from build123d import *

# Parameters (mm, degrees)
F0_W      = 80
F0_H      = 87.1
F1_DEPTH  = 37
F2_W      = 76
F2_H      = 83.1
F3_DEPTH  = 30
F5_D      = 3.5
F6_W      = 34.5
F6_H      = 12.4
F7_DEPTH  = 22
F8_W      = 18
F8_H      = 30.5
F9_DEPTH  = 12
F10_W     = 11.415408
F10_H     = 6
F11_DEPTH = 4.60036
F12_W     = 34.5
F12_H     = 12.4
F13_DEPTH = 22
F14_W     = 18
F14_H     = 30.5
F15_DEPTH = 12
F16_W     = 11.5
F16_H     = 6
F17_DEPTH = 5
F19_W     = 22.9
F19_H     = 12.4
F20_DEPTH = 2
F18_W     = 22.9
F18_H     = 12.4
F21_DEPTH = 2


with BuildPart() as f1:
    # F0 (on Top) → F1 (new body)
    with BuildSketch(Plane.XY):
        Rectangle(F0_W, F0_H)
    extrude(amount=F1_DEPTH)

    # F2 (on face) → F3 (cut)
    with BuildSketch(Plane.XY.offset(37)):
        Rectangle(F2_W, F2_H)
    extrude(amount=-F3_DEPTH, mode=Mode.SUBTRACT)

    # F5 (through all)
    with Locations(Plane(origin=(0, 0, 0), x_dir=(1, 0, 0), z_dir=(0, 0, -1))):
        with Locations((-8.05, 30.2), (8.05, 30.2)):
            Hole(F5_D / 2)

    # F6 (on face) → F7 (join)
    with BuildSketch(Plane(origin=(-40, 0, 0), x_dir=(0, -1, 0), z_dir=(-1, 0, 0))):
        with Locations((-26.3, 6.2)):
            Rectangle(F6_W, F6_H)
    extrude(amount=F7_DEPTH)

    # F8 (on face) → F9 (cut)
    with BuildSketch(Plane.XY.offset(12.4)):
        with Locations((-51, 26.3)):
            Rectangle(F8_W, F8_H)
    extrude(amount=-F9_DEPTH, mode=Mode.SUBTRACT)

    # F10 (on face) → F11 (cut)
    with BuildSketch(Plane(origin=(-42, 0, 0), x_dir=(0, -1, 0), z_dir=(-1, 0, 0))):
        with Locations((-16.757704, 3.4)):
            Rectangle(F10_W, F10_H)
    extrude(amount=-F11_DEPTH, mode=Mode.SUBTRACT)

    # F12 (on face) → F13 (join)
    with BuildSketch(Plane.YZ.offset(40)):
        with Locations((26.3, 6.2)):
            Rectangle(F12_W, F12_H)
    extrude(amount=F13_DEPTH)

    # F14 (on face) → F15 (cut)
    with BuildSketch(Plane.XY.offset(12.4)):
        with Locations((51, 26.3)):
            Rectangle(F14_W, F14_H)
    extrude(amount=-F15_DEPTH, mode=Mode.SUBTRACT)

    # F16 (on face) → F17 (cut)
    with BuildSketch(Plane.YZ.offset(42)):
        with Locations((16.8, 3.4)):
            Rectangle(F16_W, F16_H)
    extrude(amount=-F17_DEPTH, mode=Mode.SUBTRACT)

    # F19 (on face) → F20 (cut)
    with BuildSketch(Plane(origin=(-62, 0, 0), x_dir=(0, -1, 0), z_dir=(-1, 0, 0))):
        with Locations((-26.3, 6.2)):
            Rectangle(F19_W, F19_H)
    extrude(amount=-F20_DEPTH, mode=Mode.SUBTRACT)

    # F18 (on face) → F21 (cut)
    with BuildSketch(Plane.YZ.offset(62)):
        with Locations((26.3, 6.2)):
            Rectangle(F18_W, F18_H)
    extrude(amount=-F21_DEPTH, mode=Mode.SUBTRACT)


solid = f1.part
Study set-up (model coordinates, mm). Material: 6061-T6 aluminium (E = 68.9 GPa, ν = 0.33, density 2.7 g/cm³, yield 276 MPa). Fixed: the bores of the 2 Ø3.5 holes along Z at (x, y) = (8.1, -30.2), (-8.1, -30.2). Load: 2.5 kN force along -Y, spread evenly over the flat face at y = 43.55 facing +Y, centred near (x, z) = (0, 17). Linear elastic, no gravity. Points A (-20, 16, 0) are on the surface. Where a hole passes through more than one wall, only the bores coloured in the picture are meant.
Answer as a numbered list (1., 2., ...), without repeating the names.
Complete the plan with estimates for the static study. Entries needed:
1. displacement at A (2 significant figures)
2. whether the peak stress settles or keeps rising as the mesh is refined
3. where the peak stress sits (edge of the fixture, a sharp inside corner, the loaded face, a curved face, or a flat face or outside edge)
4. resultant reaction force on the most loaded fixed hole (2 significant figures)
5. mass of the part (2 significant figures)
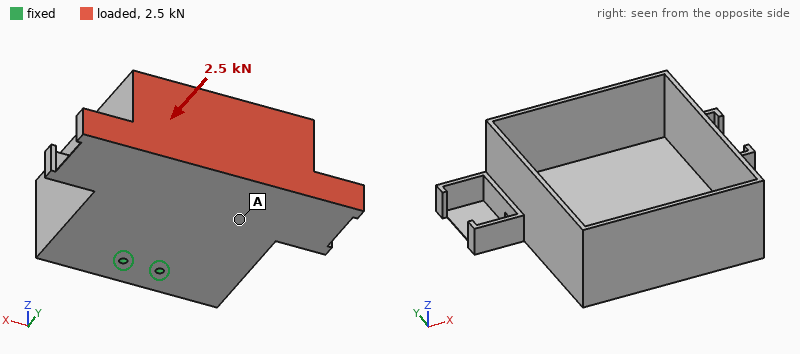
1. 0.16 mm
2. keeps rising
3. edge of the fixture
4. 1.3 kN
5. 190 g
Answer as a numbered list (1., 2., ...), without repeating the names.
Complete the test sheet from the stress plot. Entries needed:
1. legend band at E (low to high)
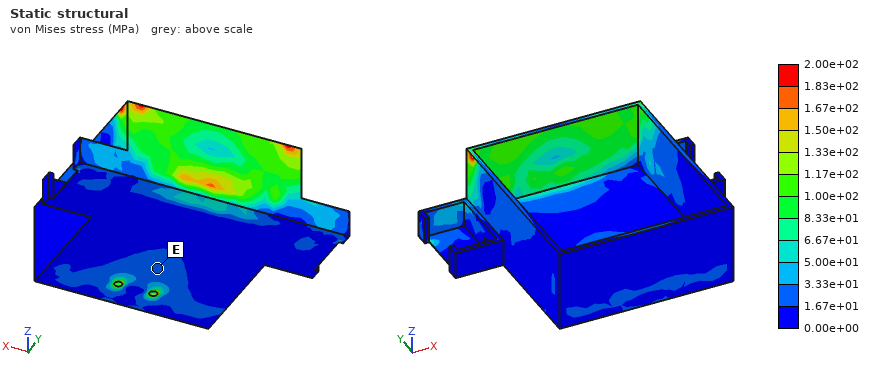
1. 1.67e+01 to 3.33e+01 MPa
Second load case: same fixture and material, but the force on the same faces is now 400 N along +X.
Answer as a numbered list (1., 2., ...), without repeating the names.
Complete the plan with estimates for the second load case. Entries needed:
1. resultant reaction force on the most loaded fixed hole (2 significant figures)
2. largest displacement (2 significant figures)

1. 1.6 kN
2. 0.10 mm
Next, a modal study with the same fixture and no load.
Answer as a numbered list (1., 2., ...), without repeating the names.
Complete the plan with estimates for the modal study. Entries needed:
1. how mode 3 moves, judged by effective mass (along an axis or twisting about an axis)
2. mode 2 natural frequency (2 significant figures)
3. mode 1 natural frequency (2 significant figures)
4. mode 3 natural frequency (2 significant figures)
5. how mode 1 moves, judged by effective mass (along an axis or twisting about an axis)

1. along X
2. 1100 Hz
3. 770 Hz
4. 2000 Hz
5. along Z
